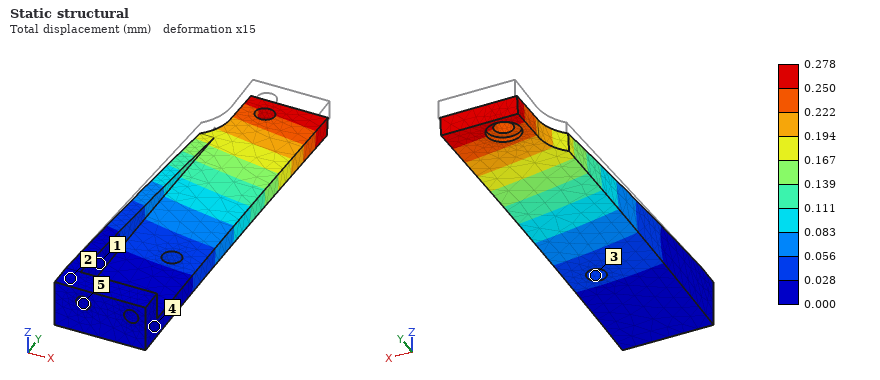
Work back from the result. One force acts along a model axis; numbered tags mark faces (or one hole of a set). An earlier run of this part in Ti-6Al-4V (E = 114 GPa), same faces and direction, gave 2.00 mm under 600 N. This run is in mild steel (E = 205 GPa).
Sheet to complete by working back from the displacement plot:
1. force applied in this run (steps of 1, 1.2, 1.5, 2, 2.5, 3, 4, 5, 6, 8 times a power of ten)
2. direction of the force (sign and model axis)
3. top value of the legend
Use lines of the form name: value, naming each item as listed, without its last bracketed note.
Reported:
force applied in this run: 150 N
direction of the force: -Z
top value of the legend: 0.278 mm
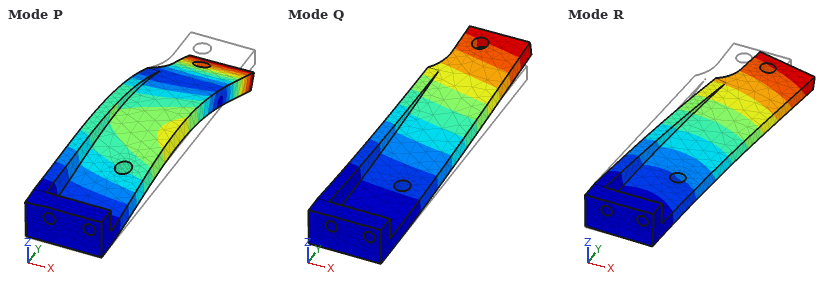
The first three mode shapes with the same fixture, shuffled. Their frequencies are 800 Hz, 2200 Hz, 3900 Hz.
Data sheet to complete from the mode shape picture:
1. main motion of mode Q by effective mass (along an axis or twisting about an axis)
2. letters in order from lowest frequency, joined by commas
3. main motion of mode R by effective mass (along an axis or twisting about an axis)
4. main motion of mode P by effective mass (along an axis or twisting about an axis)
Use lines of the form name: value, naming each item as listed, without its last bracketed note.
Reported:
main motion of mode Q by effective mass: along Z
letters in order from lowest frequency, joined by commas: Q, R, P
main motion of mode R by effective mass: along X
main motion of mode P by effective mass: along Z
